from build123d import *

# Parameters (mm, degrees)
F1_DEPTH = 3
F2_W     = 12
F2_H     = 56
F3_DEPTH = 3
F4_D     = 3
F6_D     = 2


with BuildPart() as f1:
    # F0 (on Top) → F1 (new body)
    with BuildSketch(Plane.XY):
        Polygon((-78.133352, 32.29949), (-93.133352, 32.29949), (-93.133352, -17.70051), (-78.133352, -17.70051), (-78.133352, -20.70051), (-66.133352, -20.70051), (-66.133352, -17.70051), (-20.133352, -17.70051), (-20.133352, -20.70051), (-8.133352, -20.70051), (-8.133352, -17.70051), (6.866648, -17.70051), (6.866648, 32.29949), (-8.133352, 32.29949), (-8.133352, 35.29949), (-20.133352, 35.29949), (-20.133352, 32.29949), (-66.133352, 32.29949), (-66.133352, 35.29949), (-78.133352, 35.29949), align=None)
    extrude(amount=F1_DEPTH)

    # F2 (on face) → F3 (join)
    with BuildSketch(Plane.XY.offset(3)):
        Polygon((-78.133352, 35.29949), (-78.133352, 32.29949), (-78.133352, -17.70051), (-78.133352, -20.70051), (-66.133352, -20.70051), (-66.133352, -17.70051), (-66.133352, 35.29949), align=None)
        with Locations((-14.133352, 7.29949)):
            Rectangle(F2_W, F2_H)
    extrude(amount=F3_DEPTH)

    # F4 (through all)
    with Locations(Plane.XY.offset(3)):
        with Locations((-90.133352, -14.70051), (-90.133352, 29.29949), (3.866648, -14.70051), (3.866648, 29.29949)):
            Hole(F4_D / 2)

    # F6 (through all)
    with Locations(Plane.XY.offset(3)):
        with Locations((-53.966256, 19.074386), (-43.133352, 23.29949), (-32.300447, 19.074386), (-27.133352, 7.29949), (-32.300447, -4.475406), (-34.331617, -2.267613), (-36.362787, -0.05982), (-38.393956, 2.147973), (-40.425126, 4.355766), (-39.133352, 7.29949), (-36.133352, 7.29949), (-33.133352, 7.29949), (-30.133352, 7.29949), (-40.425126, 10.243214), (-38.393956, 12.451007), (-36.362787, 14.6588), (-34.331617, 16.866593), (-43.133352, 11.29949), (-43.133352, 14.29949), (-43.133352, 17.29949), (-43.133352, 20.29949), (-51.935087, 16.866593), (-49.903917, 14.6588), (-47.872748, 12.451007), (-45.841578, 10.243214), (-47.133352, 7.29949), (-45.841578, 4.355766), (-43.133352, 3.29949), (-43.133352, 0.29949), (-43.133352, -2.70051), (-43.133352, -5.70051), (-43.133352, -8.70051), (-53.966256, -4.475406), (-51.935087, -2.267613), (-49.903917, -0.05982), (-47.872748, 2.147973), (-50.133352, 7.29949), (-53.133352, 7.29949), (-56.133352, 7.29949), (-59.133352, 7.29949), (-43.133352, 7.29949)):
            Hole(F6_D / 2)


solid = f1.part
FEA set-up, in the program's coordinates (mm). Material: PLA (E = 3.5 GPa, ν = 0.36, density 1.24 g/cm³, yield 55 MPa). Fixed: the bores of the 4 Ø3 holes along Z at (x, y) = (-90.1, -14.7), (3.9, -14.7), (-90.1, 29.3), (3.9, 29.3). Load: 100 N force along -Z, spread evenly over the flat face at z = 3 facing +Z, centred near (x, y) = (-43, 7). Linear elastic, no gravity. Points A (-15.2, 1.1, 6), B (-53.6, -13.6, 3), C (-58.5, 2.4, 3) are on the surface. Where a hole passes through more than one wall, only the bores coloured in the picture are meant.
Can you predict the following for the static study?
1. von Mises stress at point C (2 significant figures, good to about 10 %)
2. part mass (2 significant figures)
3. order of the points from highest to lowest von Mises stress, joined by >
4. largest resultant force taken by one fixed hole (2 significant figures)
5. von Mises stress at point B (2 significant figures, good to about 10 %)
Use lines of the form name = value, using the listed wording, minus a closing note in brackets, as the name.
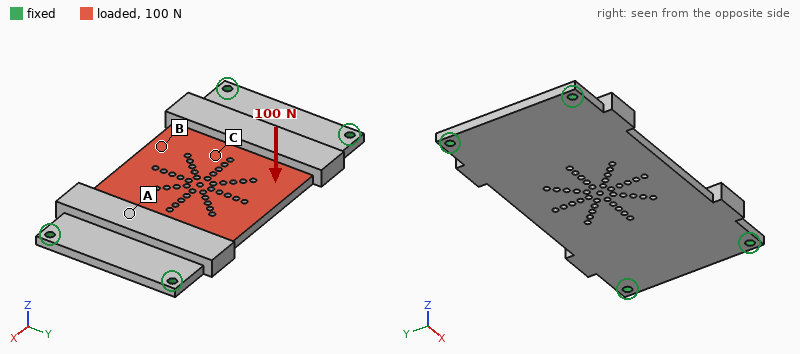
von Mises stress at point C = 6.1 MPa
part mass = 24 g
order of the points from highest to lowest von Mises stress, joined by > = B > C > A
largest resultant force taken by one fixed hole = 25 N
von Mises stress at point B = 9.7 MPa
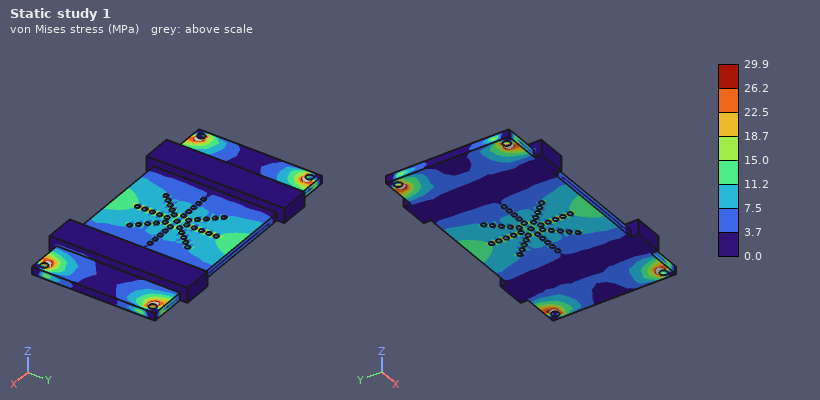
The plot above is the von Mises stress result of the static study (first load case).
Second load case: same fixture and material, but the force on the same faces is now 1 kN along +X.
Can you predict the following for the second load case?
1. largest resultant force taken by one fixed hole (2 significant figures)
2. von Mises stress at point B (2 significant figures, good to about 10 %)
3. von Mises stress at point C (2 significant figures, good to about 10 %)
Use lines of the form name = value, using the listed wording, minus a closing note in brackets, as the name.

largest resultant force taken by one fixed hole = 260 N
von Mises stress at point B = 3.6 MPa
von Mises stress at point C = 4.3 MPa
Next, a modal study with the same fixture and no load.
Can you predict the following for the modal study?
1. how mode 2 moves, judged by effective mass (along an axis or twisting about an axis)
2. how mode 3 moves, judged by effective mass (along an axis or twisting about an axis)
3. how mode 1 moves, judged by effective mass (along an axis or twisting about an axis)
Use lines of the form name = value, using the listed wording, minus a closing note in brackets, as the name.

how mode 2 moves, judged by effective mass = twisting about X
how mode 3 moves, judged by effective mass = twisting about Y
how mode 1 moves, judged by effective mass = along Z
